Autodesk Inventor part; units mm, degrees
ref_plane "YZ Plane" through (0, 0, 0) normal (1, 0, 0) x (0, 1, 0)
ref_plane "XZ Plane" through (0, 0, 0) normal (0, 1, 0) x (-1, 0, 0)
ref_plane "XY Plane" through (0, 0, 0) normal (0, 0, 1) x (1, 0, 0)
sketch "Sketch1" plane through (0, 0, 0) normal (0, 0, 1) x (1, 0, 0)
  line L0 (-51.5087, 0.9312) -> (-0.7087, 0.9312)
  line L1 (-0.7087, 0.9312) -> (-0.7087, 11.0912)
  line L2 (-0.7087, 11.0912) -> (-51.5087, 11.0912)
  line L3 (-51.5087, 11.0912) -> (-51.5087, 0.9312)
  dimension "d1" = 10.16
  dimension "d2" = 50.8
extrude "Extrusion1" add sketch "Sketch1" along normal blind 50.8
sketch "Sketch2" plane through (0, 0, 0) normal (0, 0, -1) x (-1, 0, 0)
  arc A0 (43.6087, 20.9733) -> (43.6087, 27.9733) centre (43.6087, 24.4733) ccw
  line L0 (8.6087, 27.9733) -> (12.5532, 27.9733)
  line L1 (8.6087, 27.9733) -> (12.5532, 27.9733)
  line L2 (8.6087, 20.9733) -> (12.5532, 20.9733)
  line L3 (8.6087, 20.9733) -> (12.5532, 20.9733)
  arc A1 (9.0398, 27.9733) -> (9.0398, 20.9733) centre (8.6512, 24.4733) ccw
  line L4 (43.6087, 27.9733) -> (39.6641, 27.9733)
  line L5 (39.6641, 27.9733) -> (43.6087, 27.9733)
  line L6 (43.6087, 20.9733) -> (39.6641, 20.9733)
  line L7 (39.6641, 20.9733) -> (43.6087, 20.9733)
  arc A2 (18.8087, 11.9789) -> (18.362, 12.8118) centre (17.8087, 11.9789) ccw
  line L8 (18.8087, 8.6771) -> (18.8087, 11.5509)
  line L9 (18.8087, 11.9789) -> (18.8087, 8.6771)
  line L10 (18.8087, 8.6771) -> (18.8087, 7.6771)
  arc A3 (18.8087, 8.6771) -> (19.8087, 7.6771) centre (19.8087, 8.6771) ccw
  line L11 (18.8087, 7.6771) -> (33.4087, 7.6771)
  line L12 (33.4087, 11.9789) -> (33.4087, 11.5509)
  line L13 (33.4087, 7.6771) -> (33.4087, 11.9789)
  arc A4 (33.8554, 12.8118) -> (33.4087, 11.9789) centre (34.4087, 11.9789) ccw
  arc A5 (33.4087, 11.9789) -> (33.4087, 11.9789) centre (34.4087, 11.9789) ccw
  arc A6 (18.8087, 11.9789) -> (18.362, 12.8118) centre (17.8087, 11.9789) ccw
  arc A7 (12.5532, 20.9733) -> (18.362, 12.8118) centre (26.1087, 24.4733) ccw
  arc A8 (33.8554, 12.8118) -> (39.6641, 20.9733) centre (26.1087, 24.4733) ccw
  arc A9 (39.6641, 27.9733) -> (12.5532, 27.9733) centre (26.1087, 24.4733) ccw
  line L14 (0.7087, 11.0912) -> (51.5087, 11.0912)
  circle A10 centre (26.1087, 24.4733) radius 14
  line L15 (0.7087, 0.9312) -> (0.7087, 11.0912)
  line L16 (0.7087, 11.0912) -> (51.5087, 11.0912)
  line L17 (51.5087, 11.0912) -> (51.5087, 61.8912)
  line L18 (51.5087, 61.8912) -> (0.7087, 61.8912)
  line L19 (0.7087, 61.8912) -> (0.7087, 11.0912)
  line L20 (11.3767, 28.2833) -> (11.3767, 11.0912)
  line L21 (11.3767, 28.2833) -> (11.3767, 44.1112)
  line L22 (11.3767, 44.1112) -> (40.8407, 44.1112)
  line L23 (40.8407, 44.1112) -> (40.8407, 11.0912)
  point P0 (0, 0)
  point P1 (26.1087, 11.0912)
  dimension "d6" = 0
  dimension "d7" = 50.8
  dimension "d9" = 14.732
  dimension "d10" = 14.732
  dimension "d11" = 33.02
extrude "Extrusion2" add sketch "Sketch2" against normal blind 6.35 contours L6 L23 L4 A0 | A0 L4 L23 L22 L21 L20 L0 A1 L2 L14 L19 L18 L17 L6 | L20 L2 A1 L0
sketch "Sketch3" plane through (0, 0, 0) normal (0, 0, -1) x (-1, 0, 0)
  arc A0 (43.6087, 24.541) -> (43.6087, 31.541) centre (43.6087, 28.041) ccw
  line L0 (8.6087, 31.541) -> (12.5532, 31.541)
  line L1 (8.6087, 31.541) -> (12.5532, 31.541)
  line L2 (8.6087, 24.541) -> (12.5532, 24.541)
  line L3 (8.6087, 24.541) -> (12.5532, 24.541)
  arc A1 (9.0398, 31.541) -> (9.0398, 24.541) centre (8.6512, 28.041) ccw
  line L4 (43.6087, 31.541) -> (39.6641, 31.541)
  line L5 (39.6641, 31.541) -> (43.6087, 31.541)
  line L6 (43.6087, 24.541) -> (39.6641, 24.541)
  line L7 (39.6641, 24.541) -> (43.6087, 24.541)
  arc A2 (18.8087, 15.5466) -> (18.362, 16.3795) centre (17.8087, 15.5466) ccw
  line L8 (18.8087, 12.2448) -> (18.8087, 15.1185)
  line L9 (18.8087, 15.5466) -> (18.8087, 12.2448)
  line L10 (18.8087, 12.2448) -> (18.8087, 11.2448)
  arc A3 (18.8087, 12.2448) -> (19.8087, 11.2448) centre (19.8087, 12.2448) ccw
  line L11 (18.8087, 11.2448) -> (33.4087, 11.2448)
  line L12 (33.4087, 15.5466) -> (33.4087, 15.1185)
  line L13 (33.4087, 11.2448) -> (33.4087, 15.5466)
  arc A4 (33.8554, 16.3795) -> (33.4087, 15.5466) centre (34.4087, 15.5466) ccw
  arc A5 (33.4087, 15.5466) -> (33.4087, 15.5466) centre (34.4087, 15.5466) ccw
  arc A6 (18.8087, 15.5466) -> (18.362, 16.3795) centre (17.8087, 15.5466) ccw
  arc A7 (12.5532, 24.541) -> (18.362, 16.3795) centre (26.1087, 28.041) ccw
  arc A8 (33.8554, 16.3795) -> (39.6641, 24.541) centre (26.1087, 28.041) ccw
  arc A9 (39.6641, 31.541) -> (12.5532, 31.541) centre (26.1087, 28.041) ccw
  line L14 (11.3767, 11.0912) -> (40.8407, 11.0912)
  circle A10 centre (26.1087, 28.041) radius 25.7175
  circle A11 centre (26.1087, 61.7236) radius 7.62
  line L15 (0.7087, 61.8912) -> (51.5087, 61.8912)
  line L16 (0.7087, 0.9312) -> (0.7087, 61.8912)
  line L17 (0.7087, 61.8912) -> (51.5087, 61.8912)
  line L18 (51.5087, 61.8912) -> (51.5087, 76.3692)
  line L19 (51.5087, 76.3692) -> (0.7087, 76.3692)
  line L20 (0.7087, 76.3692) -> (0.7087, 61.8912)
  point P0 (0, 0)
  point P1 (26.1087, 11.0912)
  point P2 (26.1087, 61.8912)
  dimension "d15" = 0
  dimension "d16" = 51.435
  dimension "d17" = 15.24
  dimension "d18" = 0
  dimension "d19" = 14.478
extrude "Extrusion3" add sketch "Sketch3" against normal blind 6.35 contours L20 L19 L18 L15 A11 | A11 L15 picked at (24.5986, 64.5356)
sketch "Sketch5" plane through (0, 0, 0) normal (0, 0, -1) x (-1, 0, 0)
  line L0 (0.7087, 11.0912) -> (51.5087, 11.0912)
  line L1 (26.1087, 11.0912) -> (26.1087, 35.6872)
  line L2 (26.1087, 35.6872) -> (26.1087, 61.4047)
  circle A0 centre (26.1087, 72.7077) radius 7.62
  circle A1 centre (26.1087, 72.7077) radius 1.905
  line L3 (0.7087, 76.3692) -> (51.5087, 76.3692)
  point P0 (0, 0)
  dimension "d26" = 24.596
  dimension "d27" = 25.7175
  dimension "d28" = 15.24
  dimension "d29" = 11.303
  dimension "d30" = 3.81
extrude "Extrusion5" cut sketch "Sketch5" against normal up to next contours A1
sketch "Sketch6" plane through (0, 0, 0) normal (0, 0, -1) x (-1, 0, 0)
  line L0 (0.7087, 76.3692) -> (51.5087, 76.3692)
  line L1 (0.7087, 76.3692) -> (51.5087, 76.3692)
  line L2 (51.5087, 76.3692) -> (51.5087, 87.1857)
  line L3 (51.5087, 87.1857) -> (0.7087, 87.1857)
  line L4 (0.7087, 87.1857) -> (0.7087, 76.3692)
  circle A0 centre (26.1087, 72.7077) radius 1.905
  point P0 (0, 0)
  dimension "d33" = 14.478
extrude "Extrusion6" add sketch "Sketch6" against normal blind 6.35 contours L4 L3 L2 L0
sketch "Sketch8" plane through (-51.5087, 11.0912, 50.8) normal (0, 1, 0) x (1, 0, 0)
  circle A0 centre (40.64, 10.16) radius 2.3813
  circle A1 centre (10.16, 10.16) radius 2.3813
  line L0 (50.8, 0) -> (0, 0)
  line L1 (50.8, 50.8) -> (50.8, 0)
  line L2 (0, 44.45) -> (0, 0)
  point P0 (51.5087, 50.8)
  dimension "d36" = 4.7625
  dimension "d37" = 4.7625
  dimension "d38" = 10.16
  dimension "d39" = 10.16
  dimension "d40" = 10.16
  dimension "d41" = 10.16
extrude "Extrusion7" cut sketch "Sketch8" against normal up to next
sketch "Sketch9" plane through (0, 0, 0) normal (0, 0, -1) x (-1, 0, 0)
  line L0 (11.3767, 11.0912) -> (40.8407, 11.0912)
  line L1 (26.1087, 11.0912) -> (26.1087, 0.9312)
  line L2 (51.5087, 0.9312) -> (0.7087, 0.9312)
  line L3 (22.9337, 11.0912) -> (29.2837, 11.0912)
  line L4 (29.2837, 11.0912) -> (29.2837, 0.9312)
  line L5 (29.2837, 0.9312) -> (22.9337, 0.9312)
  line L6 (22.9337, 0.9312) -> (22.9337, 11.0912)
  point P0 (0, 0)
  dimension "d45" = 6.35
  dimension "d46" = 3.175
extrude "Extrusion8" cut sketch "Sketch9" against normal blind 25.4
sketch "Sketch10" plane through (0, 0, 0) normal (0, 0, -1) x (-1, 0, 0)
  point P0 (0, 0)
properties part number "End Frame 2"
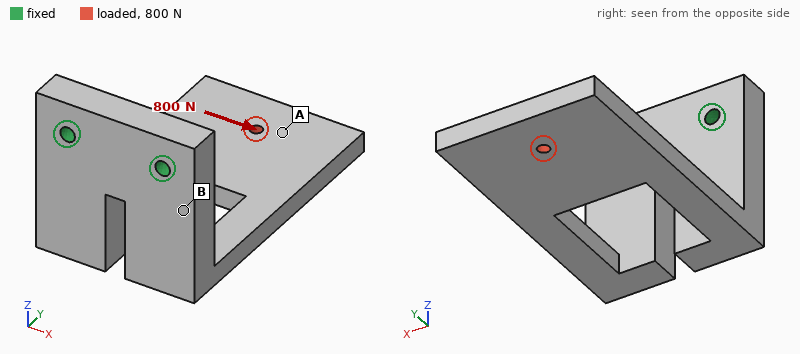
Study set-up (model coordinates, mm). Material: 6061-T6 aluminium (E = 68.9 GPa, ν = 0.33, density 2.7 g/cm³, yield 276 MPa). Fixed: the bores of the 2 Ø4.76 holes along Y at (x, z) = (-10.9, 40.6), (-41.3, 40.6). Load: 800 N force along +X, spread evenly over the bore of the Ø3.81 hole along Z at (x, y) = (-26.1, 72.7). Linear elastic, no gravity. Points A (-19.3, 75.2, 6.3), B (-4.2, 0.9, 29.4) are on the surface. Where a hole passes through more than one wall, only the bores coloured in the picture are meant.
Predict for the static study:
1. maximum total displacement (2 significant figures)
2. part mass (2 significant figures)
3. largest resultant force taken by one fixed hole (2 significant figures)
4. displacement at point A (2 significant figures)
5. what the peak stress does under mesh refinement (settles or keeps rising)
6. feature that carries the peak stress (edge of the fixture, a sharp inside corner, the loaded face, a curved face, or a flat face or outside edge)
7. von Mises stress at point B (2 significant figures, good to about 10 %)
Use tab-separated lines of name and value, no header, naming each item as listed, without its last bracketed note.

maximum total displacement	0.51 mm
part mass	110 g
largest resultant force taken by one fixed hole	1.7 kN
displacement at point A	0.42 mm
what the peak stress does under mesh refinement	keeps rising
feature that carries the peak stress	edge of the fixture
von Mises stress at point B	55 MPa
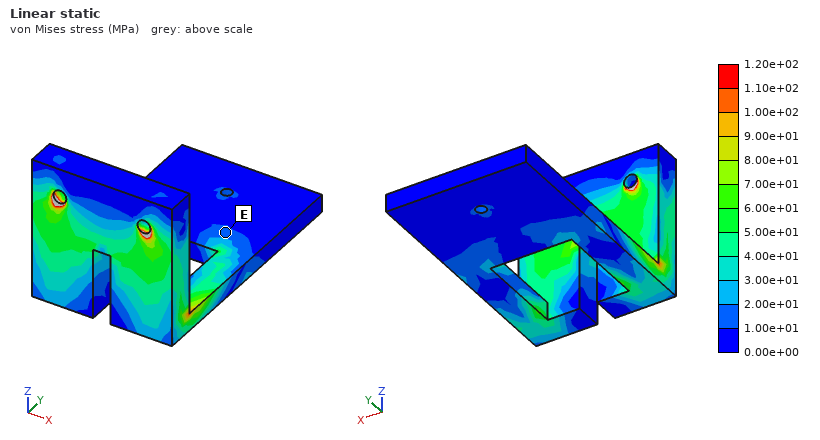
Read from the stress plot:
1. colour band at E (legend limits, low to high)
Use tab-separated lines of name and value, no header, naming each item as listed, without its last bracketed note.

colour band at E	1.00e+01 to 2.00e+01 MPa
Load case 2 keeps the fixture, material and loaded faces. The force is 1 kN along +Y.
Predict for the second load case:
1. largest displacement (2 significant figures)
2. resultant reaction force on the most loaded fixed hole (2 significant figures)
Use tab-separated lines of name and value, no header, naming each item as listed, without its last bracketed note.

largest displacement	0.24 mm
resultant reaction force on the most loaded fixed hole	500 N
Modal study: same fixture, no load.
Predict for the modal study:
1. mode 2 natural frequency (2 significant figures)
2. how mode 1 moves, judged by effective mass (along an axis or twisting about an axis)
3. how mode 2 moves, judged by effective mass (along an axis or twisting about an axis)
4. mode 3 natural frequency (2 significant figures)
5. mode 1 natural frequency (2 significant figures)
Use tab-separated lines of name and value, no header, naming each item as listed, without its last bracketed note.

mode 2 natural frequency	1200 Hz
how mode 1 moves, judged by effective mass	along Z
how mode 2 moves, judged by effective mass	along X
mode 3 natural frequency	2100 Hz
mode 1 natural frequency	500 Hz
